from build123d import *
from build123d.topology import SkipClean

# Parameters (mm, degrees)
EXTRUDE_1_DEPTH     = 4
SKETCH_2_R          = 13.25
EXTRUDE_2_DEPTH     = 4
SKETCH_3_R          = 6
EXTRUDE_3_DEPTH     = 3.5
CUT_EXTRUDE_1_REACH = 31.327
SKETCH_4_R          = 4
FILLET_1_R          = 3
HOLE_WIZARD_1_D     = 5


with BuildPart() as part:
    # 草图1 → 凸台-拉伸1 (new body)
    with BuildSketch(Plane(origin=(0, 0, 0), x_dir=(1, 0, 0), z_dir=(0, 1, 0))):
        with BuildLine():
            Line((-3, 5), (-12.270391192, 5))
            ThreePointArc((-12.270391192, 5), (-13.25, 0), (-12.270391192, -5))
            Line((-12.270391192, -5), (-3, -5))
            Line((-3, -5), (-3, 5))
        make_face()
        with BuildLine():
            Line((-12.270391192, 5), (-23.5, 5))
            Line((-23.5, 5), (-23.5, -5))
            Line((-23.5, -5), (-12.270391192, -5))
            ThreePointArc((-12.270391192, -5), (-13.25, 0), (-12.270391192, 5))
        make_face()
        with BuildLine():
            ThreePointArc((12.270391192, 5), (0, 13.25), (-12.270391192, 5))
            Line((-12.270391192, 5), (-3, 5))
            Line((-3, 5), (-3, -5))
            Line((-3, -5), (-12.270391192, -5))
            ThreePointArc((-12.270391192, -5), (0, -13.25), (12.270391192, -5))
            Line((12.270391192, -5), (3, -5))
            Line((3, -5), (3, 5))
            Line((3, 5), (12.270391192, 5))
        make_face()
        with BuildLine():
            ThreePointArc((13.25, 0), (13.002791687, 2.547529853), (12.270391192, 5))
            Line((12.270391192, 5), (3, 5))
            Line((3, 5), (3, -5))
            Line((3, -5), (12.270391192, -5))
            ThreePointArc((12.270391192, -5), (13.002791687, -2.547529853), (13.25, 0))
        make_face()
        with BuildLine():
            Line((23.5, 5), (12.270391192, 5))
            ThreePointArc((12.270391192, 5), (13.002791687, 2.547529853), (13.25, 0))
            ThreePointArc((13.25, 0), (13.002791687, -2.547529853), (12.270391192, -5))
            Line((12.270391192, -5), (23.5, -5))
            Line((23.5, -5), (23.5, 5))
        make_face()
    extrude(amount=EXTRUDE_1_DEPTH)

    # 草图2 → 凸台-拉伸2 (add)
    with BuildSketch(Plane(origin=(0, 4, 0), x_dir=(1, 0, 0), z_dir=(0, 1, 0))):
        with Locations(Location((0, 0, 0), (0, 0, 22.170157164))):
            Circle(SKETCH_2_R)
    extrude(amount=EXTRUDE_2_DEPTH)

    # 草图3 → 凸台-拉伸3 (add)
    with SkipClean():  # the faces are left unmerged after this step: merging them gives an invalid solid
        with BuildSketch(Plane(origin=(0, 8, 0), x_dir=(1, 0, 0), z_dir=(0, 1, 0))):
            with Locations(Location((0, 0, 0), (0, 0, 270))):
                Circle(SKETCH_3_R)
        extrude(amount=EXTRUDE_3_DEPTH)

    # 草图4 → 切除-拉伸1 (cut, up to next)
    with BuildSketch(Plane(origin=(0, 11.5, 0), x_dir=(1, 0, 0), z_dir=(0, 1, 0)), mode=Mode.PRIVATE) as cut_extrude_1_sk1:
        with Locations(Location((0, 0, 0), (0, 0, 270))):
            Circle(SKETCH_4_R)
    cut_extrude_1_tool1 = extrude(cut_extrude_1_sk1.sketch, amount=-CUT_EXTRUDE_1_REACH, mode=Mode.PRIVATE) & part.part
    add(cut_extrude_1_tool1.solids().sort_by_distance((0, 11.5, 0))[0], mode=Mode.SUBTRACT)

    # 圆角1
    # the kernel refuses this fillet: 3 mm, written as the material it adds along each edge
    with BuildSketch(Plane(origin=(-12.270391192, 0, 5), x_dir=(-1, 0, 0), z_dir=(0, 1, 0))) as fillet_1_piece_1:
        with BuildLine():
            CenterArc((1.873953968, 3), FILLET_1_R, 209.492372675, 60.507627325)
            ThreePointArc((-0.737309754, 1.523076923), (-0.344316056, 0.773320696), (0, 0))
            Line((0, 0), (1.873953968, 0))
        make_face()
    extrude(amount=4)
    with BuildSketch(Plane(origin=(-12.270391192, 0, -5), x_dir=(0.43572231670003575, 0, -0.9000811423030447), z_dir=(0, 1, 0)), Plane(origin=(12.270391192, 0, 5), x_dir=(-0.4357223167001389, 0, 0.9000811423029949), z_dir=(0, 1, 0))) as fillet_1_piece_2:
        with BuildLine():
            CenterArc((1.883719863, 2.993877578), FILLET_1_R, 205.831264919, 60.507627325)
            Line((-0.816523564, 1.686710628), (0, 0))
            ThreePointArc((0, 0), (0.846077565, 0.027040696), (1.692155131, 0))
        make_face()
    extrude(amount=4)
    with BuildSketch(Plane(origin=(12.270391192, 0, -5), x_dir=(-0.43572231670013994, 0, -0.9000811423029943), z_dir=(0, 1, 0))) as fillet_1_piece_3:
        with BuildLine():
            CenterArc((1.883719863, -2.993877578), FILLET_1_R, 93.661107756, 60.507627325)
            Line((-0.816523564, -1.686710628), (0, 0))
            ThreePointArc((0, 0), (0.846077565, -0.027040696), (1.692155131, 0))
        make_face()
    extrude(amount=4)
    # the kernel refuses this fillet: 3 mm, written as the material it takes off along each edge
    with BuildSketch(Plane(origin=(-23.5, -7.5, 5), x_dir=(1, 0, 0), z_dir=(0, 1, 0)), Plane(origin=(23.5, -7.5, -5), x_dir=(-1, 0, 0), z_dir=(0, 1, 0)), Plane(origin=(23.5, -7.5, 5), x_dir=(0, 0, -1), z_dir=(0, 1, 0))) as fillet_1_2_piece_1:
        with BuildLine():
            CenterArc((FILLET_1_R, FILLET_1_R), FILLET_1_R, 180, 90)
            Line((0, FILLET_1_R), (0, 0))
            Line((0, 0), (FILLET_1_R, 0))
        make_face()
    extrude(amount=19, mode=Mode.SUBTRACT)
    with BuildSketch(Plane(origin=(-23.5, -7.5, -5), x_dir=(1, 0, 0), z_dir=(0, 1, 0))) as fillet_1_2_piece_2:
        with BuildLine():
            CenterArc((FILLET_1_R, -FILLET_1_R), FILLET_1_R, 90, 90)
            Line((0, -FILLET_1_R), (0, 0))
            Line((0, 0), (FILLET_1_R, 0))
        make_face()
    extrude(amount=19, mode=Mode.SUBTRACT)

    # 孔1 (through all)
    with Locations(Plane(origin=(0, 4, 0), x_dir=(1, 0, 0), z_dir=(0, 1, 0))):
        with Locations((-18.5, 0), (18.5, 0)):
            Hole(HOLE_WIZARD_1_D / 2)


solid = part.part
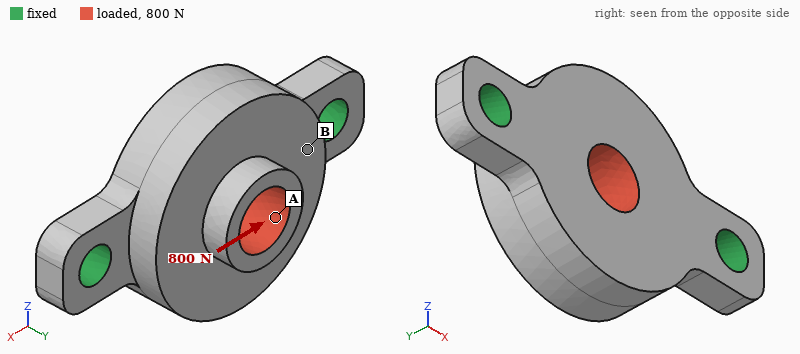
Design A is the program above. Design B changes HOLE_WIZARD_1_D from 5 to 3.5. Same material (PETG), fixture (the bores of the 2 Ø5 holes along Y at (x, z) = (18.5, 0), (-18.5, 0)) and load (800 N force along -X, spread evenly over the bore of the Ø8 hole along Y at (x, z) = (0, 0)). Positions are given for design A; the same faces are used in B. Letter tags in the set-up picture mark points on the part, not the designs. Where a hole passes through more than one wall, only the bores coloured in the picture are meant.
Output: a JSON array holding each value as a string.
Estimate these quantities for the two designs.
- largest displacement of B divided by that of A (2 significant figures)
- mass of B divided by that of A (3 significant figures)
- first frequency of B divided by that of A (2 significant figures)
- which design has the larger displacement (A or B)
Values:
["1.1", "1.02", "0.89", "B"]
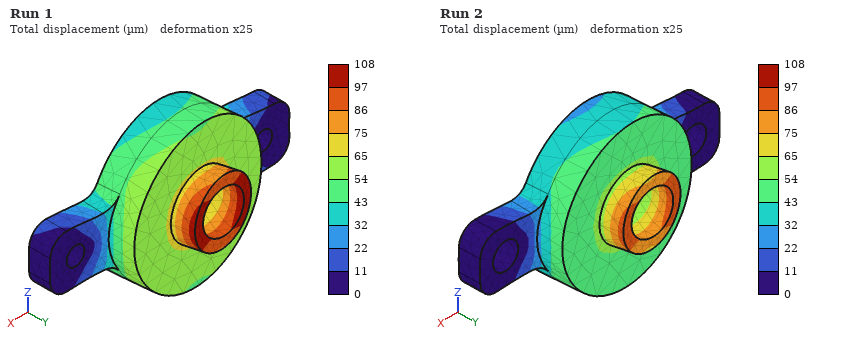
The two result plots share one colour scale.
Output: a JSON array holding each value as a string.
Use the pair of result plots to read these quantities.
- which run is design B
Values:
["Run 1"]
